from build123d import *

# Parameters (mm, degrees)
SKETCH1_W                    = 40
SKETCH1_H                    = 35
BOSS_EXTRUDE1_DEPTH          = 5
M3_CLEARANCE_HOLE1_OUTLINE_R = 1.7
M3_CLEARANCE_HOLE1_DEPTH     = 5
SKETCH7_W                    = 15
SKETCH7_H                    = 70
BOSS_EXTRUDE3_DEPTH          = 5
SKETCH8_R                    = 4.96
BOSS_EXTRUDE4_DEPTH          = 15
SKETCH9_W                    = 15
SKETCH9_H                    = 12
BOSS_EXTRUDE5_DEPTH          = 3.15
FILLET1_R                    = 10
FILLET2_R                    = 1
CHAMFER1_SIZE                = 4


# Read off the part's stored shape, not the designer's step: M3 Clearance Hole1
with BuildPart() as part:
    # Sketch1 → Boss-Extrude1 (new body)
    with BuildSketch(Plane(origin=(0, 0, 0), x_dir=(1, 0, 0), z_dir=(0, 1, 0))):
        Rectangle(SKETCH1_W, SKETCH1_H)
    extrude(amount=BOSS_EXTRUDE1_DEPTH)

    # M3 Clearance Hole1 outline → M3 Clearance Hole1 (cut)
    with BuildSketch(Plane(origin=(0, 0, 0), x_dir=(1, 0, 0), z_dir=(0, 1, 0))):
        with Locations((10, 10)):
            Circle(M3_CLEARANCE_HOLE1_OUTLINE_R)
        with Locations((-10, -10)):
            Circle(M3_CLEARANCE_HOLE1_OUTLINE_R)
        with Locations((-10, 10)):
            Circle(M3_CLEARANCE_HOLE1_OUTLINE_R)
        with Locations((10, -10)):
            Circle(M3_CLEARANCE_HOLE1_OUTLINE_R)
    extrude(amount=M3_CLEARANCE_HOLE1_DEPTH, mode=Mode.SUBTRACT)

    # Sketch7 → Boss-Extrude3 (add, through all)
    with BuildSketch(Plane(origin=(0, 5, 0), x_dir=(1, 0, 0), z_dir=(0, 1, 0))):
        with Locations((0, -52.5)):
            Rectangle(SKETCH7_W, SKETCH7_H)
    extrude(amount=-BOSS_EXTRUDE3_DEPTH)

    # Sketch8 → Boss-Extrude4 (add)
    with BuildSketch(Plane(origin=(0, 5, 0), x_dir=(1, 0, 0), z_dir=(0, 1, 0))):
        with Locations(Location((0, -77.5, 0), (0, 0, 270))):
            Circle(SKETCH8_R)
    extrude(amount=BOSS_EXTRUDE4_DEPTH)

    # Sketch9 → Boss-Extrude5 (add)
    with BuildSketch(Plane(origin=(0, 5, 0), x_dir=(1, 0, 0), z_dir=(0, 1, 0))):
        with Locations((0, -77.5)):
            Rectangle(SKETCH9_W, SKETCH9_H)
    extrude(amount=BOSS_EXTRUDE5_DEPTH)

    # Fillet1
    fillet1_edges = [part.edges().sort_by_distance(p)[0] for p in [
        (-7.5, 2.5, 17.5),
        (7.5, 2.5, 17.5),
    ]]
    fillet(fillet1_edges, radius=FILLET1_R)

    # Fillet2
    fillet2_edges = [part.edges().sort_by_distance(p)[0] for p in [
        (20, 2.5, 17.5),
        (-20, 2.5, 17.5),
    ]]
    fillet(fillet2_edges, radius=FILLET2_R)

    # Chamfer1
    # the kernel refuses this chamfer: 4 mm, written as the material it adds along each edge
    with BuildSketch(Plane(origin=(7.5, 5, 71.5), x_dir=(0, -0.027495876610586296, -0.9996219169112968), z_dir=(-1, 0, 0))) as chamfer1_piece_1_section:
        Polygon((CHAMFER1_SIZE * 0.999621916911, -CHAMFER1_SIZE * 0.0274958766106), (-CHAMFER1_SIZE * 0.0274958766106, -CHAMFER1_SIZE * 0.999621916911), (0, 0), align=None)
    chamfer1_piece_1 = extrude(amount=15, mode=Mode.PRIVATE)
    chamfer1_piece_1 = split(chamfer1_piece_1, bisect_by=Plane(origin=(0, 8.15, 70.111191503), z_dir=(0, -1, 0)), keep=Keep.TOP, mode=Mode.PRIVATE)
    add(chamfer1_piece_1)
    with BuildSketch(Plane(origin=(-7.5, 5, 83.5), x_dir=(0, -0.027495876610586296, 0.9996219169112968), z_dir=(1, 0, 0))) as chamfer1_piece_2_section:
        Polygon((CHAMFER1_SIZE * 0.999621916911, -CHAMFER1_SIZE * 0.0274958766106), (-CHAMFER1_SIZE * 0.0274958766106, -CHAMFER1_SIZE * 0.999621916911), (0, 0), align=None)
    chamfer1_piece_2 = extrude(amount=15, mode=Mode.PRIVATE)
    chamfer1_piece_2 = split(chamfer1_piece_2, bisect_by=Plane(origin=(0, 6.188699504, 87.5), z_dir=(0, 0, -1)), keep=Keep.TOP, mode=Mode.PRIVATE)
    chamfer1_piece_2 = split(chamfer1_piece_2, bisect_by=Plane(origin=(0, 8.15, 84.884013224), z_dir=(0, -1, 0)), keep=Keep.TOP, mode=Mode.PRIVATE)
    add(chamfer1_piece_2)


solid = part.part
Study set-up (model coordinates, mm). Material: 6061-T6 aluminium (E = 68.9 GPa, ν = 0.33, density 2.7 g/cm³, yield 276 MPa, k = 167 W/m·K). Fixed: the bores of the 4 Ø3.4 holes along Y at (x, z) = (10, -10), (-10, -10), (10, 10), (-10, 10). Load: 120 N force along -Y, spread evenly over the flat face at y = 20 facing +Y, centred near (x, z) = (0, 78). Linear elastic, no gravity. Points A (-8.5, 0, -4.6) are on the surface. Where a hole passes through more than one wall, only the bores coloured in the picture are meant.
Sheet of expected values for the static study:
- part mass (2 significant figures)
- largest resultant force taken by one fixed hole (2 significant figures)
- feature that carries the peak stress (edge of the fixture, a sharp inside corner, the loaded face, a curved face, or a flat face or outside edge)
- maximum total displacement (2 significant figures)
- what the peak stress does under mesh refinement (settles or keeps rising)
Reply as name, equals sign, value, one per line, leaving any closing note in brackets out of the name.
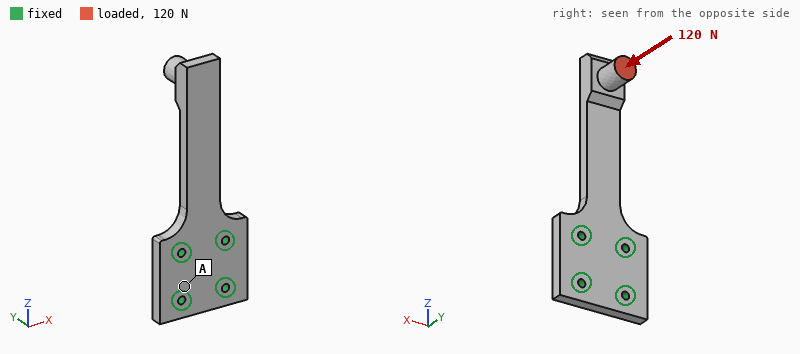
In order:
part mass = 38 g
largest resultant force taken by one fixed hole = 120 N
feature that carries the peak stress = edge of the fixture
maximum total displacement = 1.2 mm
what the peak stress does under mesh refinement = keeps rising
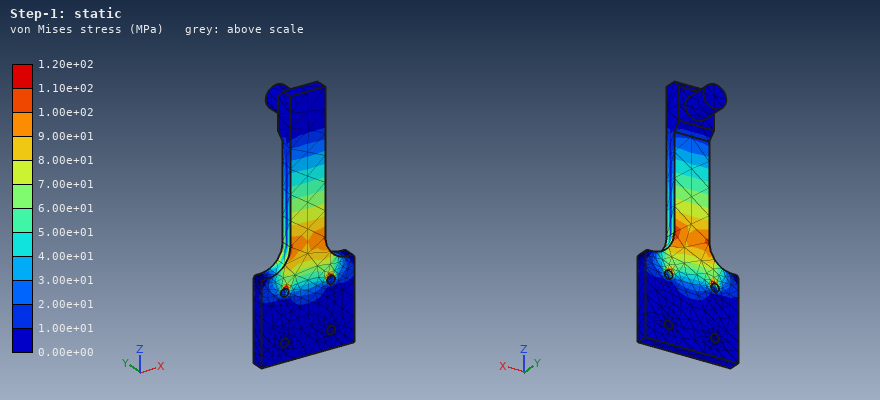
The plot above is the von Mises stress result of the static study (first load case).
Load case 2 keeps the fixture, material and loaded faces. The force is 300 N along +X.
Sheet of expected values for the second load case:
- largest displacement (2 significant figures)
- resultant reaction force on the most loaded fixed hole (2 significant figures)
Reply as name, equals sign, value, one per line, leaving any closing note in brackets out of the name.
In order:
largest displacement = 0.60 mm
resultant reaction force on the most loaded fixed hole = 870 N
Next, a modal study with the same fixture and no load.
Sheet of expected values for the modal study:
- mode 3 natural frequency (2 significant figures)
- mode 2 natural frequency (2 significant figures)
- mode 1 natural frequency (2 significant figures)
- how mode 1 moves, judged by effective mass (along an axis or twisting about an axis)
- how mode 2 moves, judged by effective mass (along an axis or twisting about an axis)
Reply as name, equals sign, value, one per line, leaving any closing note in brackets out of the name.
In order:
mode 3 natural frequency = 3800 Hz
mode 2 natural frequency = 1800 Hz
mode 1 natural frequency = 550 Hz
how mode 1 moves, judged by effective mass = along Y
how mode 2 moves, judged by effective mass = along X
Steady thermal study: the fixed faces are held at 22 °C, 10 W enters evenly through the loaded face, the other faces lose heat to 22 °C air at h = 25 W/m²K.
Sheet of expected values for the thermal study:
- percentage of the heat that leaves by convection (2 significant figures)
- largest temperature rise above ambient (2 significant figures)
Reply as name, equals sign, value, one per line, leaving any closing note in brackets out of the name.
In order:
percentage of the heat that leaves by convection = 22 %
largest temperature rise above ambient = 49 K
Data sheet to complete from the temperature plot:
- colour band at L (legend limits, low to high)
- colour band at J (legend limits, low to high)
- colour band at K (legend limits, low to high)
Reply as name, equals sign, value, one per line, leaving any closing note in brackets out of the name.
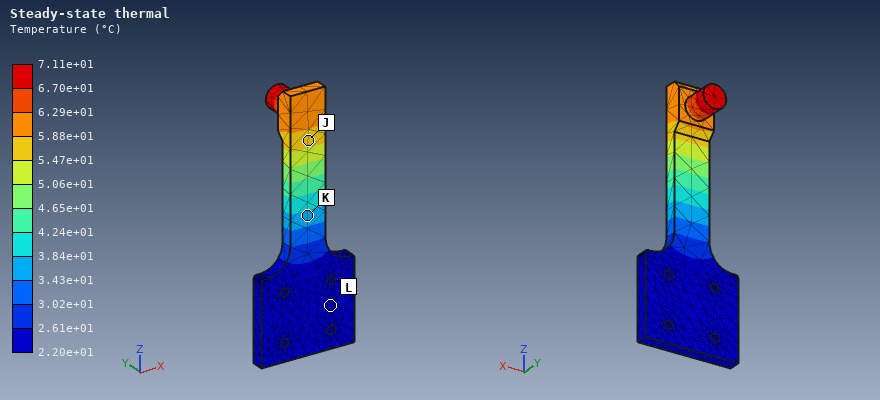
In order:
colour band at L = 2.20e+01 to 2.61e+01 °C
colour band at J = 5.47e+01 to 5.88e+01 °C
colour band at K = 3.43e+01 to 3.84e+01 °C
